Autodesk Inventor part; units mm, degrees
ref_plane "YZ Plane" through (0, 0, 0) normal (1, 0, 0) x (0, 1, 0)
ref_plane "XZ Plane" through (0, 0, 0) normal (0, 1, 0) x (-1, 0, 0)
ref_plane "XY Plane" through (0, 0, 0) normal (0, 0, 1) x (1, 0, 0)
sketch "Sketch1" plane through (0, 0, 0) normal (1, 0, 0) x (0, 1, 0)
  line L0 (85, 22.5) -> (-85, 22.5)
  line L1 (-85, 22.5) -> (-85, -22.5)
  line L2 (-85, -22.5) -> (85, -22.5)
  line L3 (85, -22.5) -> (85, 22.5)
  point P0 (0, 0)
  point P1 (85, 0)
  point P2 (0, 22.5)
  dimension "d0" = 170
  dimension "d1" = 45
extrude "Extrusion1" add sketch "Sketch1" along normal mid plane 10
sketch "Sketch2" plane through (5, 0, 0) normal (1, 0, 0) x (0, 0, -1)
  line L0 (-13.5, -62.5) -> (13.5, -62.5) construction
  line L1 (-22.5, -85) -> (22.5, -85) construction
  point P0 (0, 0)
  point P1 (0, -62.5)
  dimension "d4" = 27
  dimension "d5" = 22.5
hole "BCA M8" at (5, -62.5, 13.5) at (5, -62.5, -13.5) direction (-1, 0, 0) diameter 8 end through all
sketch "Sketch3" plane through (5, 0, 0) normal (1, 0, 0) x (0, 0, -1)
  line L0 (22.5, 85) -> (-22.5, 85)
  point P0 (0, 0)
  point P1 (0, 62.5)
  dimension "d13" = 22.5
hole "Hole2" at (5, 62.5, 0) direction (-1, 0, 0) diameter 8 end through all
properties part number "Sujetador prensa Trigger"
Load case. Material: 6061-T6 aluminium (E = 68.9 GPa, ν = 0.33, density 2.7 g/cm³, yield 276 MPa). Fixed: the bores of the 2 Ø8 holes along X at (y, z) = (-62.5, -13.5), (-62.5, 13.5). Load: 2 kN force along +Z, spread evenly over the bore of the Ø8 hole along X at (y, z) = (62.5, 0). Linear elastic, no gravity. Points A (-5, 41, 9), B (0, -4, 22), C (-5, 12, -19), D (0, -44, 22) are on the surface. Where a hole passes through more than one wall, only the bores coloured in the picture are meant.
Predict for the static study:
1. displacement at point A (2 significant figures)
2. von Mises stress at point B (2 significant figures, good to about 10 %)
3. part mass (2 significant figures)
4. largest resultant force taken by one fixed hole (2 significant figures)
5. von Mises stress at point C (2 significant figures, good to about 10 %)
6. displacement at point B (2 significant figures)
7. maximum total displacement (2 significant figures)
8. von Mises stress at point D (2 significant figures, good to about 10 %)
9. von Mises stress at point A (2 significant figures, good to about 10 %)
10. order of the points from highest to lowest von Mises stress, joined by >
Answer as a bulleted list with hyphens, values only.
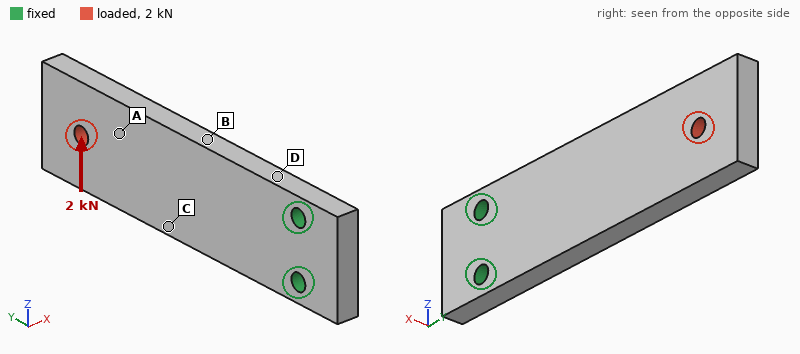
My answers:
- 0.20 mm
- 40 MPa
- 200 g
- 8.2 kN
- 25 MPa
- 0.094 mm
- 0.34 mm
- 61 MPa
- 11 MPa
- D > B > C > A
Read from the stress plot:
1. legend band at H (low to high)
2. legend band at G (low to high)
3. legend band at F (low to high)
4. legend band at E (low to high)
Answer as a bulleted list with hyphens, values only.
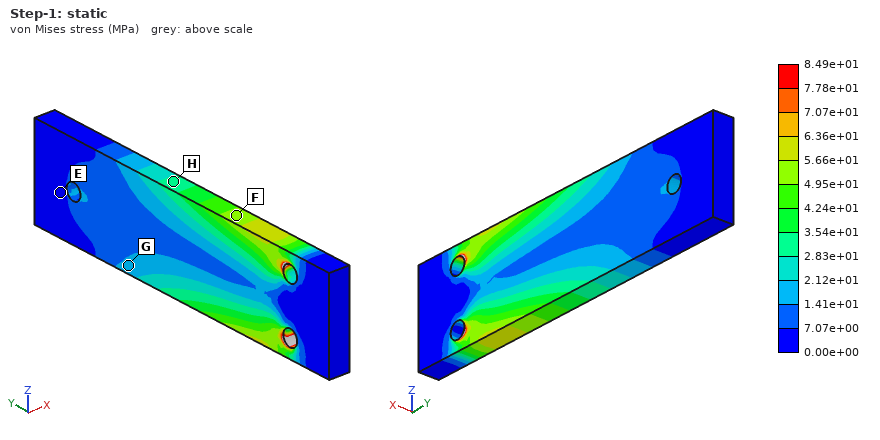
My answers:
- 2.83e+01 to 3.54e+01 MPa
- 1.41e+01 to 2.12e+01 MPa
- 4.95e+01 to 5.66e+01 MPa
- 0.00e+00 to 7.07e+00 MPa
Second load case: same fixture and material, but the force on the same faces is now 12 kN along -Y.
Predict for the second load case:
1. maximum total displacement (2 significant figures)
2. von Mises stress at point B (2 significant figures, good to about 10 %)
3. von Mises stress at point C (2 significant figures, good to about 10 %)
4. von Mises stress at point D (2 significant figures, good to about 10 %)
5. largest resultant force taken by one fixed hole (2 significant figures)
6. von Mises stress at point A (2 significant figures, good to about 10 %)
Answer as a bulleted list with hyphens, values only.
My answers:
- 57 µm
- 27 MPa
- 27 MPa
- 25 MPa
- 6.1 kN
- 30 MPa
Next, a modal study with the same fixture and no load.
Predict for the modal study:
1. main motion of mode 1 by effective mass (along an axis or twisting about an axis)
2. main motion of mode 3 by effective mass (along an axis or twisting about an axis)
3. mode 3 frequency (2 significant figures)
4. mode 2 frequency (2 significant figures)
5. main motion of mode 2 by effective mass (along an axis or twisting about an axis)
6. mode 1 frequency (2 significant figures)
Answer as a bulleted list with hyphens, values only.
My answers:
- along X
- twisting about Y
- 2300 Hz
- 1600 Hz
- along Z
- 390 Hz
